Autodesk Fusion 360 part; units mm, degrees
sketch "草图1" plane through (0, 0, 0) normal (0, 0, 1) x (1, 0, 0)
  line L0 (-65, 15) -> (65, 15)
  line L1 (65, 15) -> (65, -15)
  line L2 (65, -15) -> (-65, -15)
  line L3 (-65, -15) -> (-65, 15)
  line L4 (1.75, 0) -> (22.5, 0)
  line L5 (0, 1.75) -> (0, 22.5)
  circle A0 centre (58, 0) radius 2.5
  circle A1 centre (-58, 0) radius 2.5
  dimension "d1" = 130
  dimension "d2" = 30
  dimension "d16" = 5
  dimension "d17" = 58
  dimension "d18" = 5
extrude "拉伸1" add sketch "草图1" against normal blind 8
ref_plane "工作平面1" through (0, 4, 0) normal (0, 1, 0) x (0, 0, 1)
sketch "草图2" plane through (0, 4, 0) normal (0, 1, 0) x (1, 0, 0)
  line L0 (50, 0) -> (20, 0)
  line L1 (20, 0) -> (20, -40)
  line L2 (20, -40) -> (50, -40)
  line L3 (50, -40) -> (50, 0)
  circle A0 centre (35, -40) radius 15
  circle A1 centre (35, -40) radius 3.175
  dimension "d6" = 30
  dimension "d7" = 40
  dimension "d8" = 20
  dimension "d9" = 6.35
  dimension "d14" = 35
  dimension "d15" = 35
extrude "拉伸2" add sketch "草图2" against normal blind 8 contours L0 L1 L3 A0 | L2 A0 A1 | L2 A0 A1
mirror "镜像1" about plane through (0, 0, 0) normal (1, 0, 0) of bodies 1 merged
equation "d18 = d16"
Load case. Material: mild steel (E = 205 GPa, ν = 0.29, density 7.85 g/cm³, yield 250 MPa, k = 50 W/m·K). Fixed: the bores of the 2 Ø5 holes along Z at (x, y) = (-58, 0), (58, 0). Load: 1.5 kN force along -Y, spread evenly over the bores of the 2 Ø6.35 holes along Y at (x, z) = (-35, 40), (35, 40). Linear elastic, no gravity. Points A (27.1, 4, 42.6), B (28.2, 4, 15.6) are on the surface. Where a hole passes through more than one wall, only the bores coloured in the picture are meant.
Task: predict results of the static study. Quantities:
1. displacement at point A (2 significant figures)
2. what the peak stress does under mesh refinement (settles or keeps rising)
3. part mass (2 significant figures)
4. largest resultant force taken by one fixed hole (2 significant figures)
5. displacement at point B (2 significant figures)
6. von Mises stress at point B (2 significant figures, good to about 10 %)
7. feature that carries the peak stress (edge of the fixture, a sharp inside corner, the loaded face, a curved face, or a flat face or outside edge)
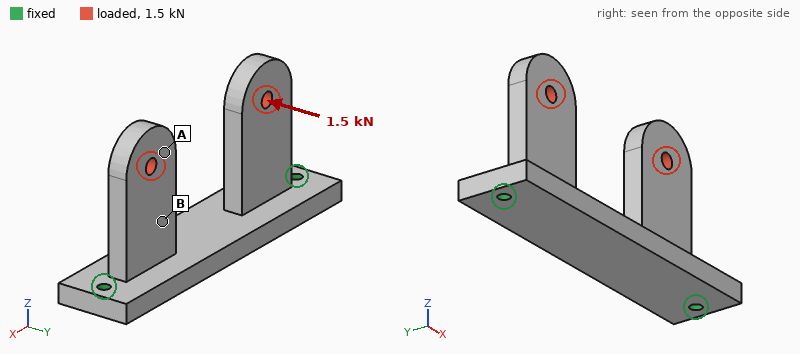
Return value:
0.16 mm
keeps rising
430 g
750 N
0.057 mm
54 MPa
edge of the fixture
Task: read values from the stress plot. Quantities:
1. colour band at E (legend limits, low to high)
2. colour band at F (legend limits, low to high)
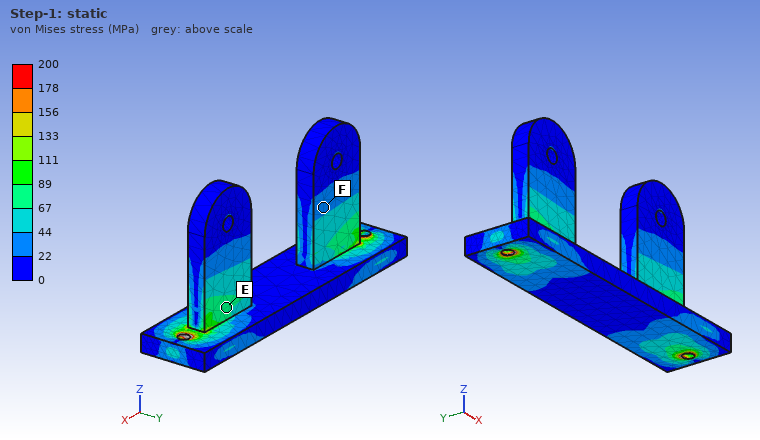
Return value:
67 to 89 MPa
22 to 44 MPa
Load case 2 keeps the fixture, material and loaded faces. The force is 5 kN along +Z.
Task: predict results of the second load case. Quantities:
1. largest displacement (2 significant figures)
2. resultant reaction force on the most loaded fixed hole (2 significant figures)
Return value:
0.10 mm
2.5 kN
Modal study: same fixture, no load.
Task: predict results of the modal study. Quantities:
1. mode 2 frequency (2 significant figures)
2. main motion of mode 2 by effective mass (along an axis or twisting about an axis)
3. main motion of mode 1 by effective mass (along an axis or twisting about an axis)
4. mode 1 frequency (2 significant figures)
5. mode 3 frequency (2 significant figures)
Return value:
1700 Hz
along Z
along Y
1500 Hz
1800 Hz
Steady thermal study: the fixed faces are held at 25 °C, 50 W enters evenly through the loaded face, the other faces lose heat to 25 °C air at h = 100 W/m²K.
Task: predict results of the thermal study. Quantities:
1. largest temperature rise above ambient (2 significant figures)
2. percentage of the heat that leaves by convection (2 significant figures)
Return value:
66 K
75 %
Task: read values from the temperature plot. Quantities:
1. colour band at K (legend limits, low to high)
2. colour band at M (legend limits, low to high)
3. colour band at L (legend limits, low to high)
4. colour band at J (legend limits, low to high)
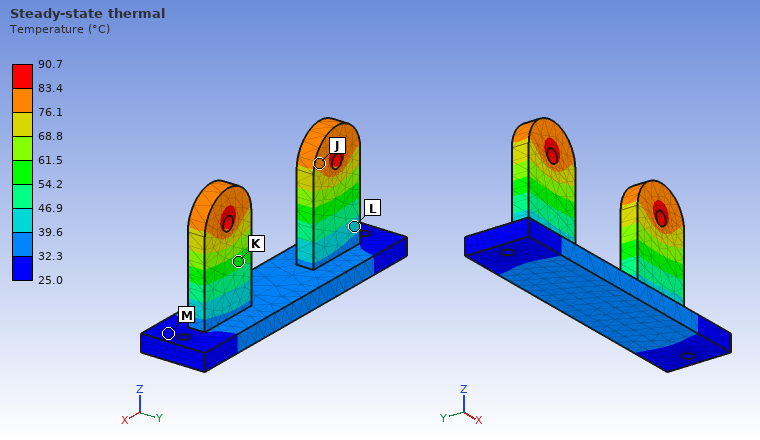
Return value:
54.2 to 61.5 °C
25.0 to 32.3 °C
39.6 to 46.9 °C
76.1 to 83.4 °C
